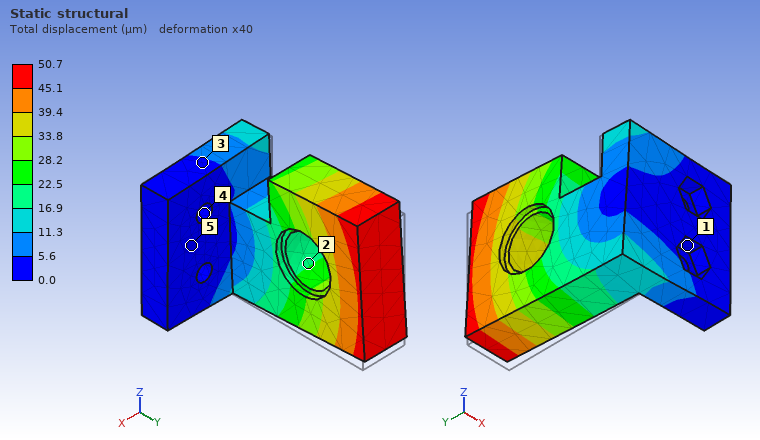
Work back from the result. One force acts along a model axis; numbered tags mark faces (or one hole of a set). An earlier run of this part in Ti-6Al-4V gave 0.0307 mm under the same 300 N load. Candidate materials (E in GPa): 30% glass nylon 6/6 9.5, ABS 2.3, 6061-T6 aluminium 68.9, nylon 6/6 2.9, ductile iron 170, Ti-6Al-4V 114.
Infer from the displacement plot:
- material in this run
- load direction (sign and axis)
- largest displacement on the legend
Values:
6061-T6 aluminium
+Z
50.7 µm
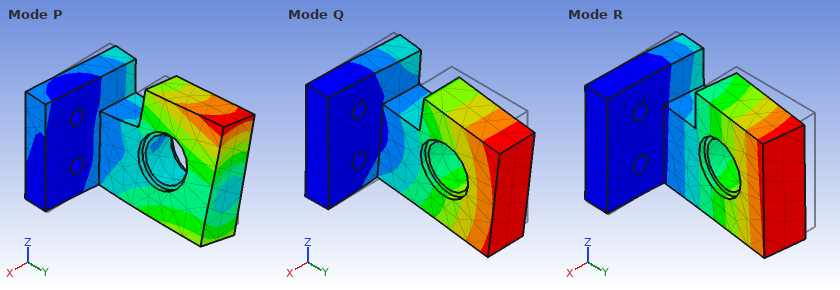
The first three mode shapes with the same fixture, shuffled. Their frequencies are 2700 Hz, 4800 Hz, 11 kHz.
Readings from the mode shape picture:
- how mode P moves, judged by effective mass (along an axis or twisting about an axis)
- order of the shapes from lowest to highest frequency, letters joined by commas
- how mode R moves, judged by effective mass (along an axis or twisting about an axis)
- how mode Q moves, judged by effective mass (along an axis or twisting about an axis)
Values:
along Y
R, Q, P
along X
along Z
